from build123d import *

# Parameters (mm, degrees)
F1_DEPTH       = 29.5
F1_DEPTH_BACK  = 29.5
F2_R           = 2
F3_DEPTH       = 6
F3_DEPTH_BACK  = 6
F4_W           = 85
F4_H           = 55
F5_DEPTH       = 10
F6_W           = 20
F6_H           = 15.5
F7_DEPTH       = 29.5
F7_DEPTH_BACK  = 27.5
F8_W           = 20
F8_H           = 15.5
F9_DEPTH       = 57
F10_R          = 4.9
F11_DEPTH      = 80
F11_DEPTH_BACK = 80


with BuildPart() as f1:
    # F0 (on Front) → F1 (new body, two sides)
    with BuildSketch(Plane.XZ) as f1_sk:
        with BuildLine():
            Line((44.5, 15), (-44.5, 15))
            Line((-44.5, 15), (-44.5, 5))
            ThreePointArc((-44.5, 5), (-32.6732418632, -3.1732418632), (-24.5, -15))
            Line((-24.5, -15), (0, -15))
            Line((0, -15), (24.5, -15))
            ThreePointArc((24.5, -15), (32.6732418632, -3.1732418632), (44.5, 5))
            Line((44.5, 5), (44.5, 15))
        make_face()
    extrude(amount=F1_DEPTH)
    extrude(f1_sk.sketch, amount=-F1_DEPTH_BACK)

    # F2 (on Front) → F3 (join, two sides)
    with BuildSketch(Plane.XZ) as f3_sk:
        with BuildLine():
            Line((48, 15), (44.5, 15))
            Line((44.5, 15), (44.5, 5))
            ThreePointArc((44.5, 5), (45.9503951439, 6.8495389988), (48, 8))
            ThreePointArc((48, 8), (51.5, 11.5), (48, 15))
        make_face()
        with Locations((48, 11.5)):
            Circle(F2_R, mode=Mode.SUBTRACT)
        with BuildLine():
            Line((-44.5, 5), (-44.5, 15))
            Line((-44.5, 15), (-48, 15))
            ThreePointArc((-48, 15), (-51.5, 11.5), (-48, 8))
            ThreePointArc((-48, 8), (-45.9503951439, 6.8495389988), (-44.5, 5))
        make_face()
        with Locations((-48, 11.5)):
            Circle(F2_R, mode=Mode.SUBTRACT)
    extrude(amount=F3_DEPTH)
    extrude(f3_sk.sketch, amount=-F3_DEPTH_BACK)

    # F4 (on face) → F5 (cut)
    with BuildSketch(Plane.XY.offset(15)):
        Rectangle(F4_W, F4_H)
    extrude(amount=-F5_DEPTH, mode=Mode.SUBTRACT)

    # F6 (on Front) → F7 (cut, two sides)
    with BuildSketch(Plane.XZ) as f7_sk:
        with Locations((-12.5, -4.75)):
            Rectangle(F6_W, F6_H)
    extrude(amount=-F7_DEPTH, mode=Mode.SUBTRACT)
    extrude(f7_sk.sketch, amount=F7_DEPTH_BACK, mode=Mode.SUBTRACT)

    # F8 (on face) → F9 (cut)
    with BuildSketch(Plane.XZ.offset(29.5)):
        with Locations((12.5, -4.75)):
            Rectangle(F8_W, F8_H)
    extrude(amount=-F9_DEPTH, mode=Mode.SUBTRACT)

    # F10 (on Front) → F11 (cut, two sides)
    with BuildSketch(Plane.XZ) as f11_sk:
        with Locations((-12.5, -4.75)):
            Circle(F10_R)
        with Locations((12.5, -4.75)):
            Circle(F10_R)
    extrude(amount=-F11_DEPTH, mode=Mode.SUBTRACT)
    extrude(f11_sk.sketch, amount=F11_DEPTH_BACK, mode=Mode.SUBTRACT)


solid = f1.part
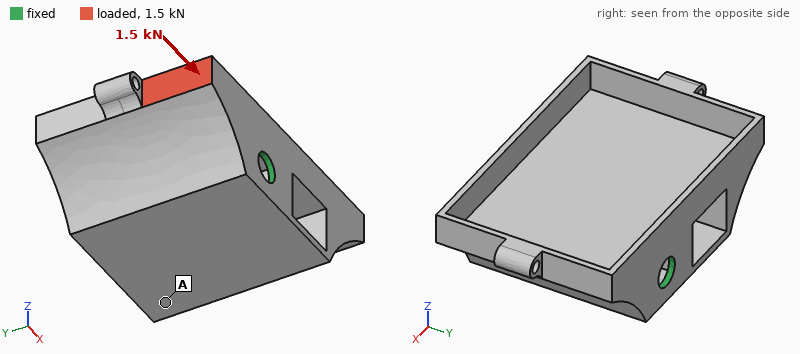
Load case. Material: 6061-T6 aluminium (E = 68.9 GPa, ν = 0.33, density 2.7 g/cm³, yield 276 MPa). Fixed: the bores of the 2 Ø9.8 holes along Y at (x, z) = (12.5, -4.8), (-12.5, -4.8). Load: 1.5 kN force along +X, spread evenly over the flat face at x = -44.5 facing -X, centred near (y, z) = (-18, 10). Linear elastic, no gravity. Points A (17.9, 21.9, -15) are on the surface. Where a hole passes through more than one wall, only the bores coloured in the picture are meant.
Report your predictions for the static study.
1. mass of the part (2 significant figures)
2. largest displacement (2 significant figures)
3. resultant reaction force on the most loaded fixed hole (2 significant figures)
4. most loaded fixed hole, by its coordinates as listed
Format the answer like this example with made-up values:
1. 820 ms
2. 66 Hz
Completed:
1. 130 g
2. 0.27 mm
3. 1.2 kN
4. (-12.5, -4.8)
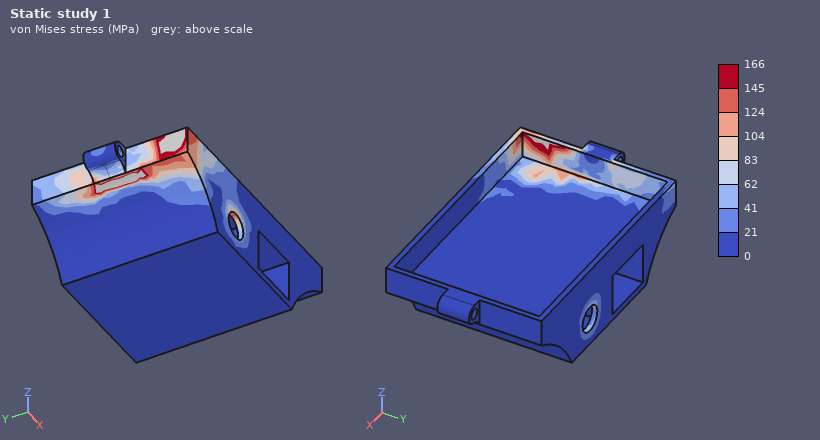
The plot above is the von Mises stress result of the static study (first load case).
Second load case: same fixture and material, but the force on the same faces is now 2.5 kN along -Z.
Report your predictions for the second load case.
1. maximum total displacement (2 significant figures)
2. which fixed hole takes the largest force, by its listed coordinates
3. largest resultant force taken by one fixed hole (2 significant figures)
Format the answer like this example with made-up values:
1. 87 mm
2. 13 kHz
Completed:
1. 0.39 mm
2. (-12.5, -4.8)
3. 2.2 kN
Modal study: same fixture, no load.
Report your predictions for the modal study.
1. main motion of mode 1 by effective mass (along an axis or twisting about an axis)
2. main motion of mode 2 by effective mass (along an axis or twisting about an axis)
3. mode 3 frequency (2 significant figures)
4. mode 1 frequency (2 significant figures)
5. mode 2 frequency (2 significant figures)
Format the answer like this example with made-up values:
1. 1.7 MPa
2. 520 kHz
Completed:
1. twisting about Y
2. along Z
3. 5700 Hz
4. 2700 Hz
5. 4100 Hz
